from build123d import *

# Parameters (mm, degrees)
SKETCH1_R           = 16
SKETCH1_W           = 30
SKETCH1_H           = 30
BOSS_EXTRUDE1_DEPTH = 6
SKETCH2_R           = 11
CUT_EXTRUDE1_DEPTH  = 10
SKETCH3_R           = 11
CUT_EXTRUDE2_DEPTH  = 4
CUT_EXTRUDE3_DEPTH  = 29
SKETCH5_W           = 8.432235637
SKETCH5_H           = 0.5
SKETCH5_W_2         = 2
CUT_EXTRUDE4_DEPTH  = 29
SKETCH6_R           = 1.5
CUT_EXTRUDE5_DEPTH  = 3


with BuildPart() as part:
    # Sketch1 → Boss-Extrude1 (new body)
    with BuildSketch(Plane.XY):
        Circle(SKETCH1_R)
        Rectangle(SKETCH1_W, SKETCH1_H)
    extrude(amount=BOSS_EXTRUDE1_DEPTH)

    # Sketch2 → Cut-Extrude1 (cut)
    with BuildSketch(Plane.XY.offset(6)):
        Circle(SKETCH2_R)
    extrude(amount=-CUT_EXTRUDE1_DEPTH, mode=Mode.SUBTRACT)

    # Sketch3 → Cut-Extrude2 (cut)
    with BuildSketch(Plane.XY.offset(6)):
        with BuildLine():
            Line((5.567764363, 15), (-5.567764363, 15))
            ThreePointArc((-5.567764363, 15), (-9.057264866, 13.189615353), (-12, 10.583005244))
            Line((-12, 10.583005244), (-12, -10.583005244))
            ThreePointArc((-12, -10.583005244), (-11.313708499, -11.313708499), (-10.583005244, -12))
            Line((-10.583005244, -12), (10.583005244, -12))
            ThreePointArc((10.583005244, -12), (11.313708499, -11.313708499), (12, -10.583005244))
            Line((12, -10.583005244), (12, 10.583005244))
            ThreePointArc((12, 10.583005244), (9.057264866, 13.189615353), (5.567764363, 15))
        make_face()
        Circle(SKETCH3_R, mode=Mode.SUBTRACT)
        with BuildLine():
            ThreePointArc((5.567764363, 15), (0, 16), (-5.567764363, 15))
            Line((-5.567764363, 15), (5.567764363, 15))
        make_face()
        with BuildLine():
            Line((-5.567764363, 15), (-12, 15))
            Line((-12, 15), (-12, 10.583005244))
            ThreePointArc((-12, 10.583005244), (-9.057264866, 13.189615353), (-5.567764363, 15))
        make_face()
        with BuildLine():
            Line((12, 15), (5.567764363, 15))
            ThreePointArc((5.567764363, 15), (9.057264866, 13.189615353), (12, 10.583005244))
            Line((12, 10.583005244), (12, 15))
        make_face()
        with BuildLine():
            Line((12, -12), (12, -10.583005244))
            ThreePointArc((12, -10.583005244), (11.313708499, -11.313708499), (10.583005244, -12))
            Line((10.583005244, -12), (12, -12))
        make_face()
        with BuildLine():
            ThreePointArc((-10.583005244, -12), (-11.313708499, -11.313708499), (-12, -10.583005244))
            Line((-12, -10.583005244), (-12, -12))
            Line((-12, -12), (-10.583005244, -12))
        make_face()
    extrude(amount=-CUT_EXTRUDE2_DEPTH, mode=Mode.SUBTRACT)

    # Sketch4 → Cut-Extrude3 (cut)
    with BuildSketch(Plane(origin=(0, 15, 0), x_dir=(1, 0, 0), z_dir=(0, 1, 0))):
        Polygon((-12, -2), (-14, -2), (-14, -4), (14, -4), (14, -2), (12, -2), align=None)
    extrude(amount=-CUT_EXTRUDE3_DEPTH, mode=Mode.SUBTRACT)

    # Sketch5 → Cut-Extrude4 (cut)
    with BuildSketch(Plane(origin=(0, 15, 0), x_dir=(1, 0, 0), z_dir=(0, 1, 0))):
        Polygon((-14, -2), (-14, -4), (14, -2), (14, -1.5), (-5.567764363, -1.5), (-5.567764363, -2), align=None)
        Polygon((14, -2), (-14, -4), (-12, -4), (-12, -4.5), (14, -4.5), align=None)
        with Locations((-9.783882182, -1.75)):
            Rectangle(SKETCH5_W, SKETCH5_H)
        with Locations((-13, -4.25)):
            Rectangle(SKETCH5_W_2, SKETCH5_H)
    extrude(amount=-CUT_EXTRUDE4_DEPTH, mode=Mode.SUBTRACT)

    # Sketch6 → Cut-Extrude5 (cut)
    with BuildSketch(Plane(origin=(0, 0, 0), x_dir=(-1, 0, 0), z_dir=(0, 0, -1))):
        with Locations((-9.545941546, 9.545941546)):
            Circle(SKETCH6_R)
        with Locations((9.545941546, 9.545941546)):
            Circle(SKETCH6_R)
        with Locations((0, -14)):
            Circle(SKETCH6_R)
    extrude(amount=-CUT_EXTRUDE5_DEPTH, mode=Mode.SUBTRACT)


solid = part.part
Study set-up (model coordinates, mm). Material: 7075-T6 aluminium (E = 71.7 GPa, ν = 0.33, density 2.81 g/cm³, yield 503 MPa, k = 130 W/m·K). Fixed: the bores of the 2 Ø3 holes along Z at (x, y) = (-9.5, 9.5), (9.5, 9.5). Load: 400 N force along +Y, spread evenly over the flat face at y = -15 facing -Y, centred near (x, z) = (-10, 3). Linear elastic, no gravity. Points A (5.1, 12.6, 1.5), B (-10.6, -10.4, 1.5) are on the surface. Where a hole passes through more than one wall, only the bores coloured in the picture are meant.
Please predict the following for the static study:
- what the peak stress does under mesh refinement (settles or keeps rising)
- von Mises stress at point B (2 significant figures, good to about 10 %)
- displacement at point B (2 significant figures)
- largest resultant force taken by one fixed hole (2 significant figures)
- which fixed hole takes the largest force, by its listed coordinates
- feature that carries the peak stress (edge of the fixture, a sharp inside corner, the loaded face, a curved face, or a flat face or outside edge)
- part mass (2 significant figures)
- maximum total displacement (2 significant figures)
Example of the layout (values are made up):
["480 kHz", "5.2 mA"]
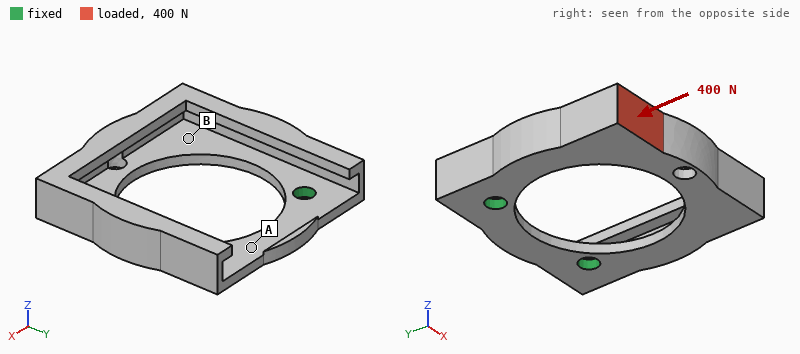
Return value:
["keeps rising", "31 MPa", "0.13 mm", "380 N", "(-9.5, 9.5)", "edge of the fixture", "4.3 g", "0.19 mm"]
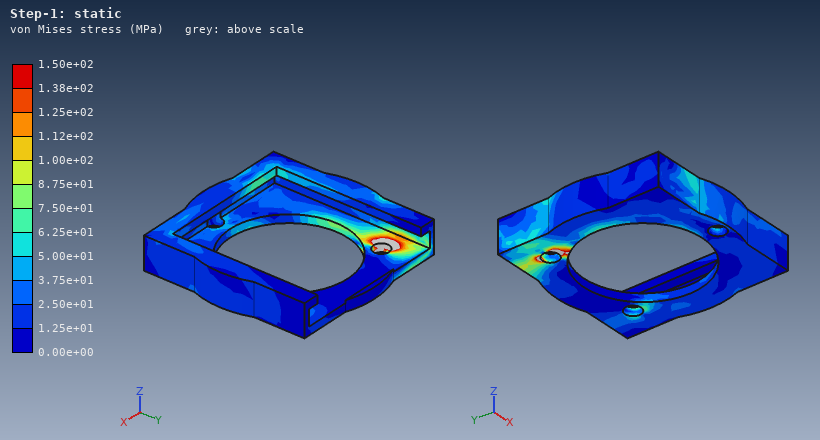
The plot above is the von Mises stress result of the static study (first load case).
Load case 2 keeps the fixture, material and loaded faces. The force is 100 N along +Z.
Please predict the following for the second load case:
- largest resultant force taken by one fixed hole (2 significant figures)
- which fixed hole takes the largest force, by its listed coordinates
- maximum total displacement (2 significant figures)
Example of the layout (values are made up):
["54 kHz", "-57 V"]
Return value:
["89 N", "(-9.5, 9.5)", "0.53 mm"]
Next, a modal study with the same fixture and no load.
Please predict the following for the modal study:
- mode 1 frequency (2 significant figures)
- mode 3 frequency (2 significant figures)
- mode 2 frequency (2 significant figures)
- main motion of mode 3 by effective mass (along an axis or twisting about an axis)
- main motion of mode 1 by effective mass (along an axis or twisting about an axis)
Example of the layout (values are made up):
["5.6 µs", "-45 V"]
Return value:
["2100 Hz", "6500 Hz", "3400 Hz", "along X", "along Z"]
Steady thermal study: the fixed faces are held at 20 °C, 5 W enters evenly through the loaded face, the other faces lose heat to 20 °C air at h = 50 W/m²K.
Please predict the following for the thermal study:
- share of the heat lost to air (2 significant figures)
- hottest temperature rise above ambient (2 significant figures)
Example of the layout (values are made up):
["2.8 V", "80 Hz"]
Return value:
["30 %", "32 K"]
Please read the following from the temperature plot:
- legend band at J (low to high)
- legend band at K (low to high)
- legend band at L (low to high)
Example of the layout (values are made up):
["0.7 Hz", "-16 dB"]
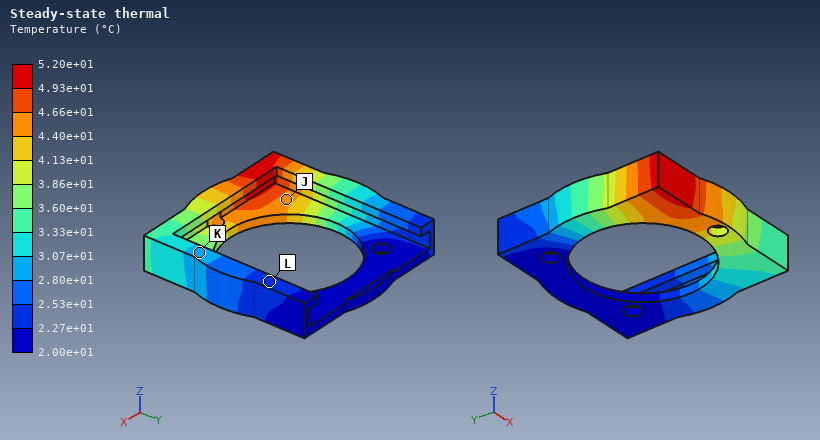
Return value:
["4.40e+01 to 4.66e+01 °C", "2.80e+01 to 3.07e+01 °C", "2.27e+01 to 2.53e+01 °C"]
